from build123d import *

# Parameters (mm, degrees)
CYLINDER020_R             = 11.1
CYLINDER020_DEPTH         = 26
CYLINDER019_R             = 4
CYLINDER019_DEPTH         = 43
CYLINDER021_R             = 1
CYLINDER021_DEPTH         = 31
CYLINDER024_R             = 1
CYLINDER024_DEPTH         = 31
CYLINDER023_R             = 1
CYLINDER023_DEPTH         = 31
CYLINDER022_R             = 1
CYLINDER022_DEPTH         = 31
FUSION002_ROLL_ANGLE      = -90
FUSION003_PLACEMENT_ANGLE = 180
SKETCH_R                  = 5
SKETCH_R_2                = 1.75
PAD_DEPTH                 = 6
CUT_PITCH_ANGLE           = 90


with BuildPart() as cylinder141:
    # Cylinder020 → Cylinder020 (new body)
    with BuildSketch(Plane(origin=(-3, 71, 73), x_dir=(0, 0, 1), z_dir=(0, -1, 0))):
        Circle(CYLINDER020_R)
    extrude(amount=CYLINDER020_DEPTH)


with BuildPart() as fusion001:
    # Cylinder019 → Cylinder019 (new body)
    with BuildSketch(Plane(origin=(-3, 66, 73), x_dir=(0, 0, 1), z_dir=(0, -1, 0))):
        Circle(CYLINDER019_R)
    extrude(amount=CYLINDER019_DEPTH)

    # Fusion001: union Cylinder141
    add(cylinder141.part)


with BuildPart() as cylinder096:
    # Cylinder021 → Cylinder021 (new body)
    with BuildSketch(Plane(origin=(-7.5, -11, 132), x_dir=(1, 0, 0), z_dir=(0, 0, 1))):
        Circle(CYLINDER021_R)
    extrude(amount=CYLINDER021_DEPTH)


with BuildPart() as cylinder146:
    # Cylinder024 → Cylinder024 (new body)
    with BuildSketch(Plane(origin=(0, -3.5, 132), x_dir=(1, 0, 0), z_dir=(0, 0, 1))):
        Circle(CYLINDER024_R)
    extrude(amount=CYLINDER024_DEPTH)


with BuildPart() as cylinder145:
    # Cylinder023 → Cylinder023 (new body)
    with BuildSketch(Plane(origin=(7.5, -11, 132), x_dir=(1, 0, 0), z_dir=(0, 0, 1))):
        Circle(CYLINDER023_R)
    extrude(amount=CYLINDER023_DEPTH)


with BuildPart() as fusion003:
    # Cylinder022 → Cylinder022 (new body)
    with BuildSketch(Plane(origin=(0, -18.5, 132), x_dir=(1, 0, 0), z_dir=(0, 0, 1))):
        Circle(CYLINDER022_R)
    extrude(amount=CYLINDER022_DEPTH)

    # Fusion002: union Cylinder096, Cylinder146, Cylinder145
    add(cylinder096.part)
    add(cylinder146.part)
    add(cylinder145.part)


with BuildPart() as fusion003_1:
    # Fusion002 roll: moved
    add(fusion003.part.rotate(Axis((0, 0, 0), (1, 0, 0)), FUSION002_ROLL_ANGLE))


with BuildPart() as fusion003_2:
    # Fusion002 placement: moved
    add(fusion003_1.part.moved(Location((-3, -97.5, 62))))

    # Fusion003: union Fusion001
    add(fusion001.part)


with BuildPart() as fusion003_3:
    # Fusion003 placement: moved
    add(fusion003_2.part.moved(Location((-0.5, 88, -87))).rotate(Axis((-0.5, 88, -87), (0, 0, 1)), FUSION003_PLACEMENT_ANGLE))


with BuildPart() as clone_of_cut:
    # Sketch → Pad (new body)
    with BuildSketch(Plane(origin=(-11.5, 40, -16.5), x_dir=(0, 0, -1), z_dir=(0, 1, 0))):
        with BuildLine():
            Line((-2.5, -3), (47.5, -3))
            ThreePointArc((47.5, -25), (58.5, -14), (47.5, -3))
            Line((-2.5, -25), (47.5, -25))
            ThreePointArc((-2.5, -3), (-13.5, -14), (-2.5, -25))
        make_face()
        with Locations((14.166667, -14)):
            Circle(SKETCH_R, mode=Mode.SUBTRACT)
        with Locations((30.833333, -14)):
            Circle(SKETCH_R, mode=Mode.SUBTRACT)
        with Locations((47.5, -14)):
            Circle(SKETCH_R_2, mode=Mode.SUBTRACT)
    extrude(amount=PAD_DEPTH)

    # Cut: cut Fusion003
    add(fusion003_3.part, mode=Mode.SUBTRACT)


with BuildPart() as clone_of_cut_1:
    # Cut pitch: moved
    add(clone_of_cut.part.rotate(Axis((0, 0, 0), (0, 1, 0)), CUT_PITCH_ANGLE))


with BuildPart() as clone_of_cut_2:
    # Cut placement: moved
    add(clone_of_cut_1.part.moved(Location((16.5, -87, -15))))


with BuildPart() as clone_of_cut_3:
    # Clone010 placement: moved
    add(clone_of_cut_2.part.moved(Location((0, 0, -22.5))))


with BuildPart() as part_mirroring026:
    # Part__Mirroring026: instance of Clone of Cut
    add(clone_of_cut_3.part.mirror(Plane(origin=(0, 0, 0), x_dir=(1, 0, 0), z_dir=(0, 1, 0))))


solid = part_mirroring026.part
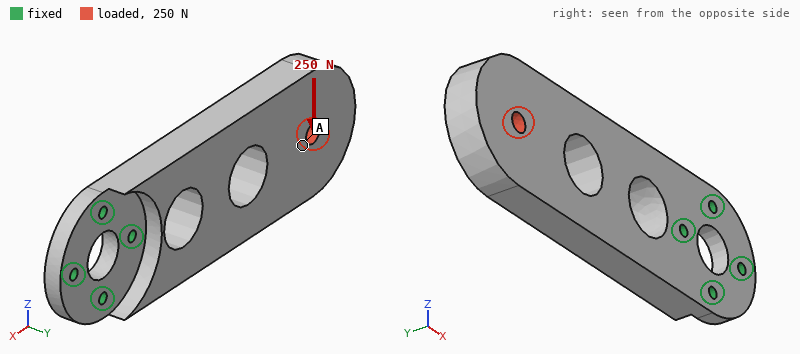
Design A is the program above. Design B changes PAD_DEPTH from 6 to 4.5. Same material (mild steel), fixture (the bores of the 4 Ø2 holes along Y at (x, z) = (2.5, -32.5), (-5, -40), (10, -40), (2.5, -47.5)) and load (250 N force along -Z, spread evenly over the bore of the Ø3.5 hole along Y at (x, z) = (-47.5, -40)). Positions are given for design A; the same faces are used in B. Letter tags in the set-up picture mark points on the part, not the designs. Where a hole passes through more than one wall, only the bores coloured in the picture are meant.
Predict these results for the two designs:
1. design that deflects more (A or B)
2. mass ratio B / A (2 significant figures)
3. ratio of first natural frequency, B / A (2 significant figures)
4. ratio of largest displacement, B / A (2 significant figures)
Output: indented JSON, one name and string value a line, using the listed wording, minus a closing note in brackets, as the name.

{
  "design that deflects more": "B",
  "mass ratio B / A": "0.71",
  "ratio of first natural frequency, B / A": "0.64",
  "ratio of largest displacement, B / A": "1.7"
}
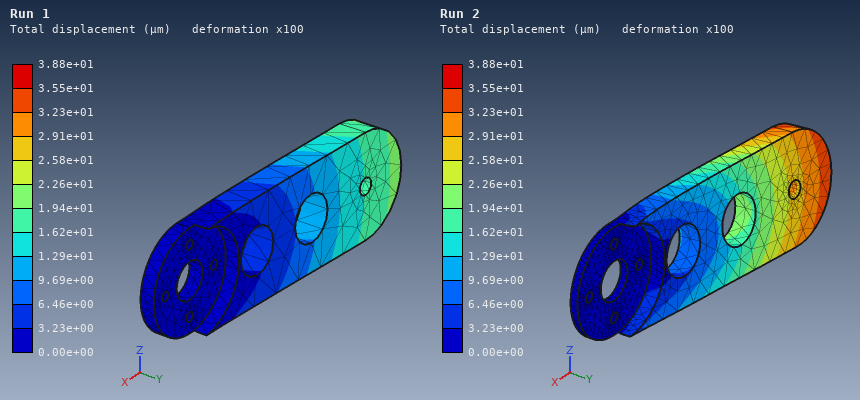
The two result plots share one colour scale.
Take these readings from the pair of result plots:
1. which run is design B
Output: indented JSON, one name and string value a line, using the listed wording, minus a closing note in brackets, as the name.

{
  "which run is design B": "Run 2"
}
